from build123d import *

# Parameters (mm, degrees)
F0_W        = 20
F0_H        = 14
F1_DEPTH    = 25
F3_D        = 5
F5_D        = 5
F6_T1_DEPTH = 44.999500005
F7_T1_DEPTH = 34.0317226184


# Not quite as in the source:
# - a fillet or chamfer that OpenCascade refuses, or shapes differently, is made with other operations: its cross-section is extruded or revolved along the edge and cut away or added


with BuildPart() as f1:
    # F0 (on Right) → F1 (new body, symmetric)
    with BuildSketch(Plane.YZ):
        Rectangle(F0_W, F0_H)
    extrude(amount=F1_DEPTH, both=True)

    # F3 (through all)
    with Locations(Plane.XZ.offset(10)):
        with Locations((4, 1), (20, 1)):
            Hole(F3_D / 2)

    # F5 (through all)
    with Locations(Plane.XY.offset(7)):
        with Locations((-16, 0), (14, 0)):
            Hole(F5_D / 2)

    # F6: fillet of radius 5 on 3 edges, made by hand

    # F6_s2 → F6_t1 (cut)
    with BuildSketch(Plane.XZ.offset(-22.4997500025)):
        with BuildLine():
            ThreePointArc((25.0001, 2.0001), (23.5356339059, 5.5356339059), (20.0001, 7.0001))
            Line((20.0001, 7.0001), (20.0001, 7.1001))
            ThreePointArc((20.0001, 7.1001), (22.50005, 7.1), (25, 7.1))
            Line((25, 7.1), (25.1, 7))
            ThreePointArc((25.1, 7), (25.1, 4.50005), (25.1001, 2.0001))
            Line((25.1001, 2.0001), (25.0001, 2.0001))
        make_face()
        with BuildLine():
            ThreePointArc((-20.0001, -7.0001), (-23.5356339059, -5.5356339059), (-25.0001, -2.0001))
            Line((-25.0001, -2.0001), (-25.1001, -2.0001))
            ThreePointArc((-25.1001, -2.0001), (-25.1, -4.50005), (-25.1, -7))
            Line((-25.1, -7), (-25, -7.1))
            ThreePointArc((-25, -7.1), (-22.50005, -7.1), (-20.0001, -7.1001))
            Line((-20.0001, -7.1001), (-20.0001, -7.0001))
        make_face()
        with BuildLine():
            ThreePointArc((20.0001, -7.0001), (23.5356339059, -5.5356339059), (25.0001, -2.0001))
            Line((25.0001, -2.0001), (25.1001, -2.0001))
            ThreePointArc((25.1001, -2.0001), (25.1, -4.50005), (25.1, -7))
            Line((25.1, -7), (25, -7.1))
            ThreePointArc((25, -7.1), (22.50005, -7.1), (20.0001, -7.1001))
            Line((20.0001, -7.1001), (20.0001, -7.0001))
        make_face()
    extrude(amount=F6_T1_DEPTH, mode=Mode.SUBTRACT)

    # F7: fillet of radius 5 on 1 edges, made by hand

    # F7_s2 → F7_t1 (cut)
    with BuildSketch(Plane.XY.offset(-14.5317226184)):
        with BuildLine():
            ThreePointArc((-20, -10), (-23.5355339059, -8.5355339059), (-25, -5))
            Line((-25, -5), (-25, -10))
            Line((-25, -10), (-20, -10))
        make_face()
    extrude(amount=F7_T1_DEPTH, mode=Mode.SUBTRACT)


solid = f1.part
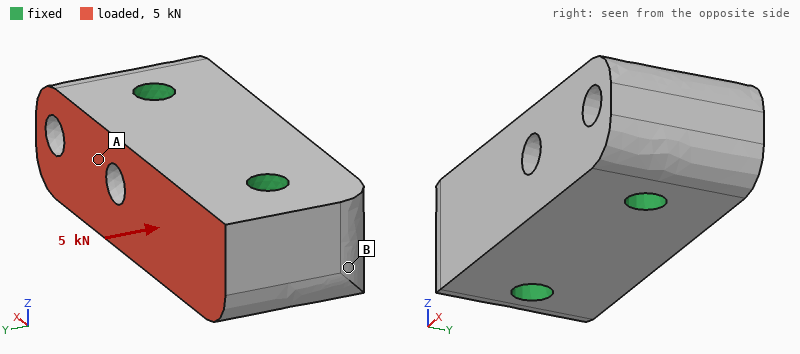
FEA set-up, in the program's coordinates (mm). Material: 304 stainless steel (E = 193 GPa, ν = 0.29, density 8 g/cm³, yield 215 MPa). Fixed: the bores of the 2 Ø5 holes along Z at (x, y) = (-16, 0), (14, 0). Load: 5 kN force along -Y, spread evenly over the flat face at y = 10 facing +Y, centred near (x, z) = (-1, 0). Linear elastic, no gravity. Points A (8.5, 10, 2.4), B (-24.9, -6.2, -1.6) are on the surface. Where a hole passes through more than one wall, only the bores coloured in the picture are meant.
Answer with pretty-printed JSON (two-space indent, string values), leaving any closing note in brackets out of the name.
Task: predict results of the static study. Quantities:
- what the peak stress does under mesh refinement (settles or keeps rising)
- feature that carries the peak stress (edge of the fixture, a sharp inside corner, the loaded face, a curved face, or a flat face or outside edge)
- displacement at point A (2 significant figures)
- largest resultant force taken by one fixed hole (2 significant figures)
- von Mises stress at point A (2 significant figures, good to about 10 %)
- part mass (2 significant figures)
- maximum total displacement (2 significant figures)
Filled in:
{
  "what the peak stress does under mesh refinement": "keeps rising",
  "feature that carries the peak stress": "edge of the fixture",
  "displacement at point A": "0.69 µm",
  "largest resultant force taken by one fixed hole": "2.5 kN",
  "von Mises stress at point A": "9.0 MPa",
  "part mass": "98 g",
  "maximum total displacement": "1.1 µm"
}
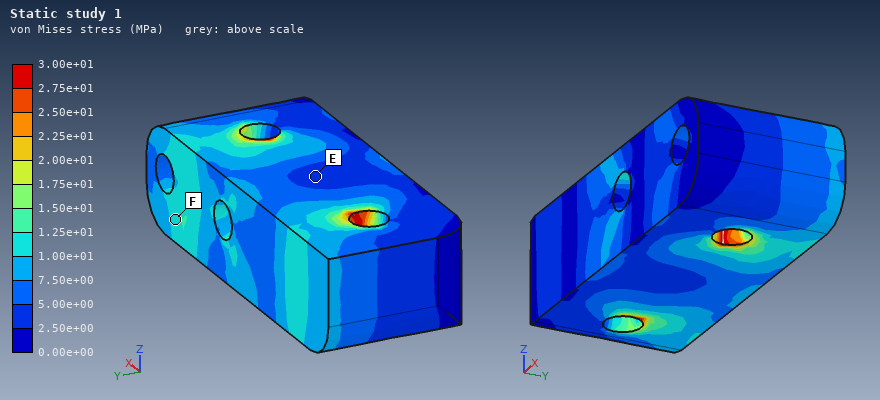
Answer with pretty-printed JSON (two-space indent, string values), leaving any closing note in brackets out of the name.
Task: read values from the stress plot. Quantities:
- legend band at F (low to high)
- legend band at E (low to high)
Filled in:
{
  "legend band at F": "1.00e+01 to 1.25e+01 MPa",
  "legend band at E": "2.50e+00 to 5.00e+00 MPa"
}
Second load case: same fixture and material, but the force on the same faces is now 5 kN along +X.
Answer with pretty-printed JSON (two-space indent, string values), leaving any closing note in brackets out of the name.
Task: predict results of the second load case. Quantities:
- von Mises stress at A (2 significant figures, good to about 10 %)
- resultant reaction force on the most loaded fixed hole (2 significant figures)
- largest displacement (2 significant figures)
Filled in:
{
  "von Mises stress at A": "15 MPa",
  "resultant reaction force on the most loaded fixed hole": "2.9 kN",
  "largest displacement": "3.2 µm"
}
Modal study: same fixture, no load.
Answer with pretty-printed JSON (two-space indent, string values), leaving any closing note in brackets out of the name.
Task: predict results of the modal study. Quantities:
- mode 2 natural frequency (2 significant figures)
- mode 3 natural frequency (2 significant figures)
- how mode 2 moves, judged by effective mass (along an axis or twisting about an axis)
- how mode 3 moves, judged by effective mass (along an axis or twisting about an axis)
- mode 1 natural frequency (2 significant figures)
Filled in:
{
  "mode 2 natural frequency": "38 kHz",
  "mode 3 natural frequency": "40 kHz",
  "how mode 2 moves, judged by effective mass": "along Z",
  "how mode 3 moves, judged by effective mass": "twisting about X",
  "mode 1 natural frequency": "36 kHz"
}
